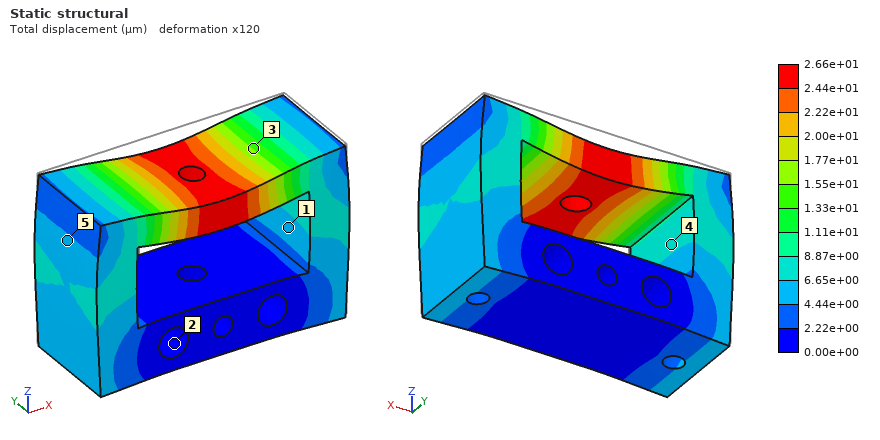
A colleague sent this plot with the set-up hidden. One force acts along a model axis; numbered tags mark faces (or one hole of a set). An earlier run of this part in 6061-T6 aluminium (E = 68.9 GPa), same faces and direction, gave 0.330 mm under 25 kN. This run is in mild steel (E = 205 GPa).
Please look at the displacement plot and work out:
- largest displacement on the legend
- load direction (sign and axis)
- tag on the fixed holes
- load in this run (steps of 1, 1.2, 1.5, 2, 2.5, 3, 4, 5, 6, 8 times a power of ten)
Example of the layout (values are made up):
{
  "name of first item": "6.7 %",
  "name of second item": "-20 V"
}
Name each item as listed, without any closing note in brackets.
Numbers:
{
  "largest displacement on the legend": "2.66e+01 µm",
  "load direction": "-Z",
  "tag on the fixed holes": "2",
  "load in this run": "6 kN"
}
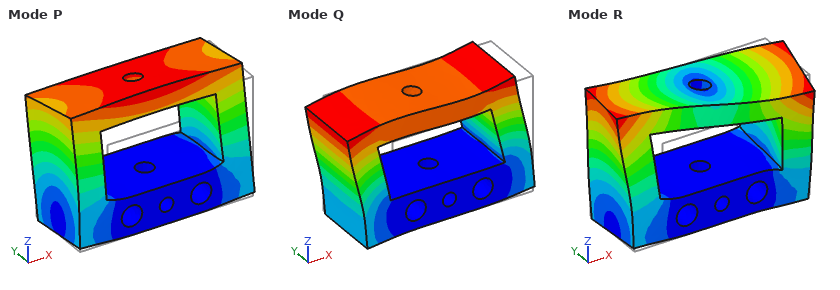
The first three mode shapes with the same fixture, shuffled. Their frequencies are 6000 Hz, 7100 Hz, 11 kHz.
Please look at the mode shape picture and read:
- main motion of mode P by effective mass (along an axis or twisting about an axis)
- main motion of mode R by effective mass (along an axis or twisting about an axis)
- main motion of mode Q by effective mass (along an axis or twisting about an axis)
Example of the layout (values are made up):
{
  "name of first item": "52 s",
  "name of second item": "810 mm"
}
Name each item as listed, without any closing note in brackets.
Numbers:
{
  "main motion of mode P by effective mass": "along Y",
  "main motion of mode R by effective mass": "twisting about Z",
  "main motion of mode Q by effective mass": "along X"
}
